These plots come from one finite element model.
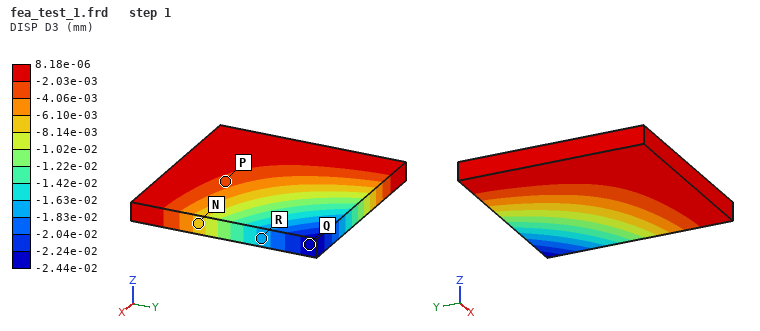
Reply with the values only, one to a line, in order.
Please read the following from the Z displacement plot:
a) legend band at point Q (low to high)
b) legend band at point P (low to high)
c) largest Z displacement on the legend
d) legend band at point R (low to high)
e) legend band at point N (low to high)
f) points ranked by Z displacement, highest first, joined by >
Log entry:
-2.44e-02 to -2.24e-02 mm
-4.06e-03 to -2.03e-03 mm
8.18e-06 mm
-1.83e-02 to -1.63e-02 mm
-8.14e-03 to -6.10e-03 mm
P > N > R > Q
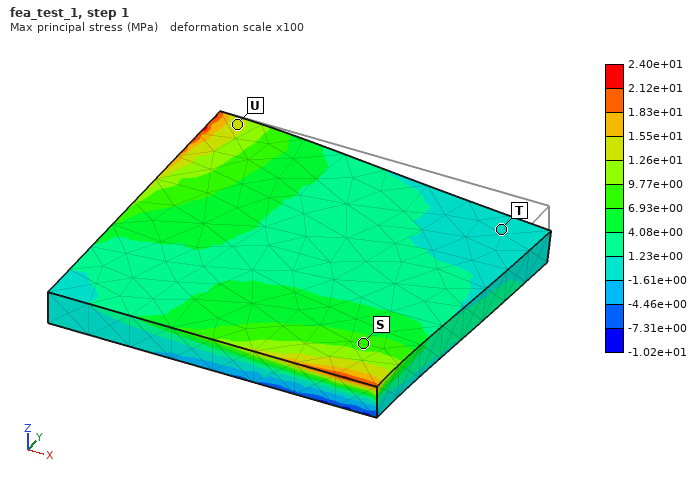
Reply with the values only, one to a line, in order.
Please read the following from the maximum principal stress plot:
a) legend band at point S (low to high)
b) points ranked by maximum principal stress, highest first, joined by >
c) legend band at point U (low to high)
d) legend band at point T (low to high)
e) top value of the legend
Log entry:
6.93e+00 to 9.77e+00 MPa
U > S > T
1.26e+01 to 1.55e+01 MPa
-1.61e+00 to 1.23e+00 MPa
2.40e+01 MPa
